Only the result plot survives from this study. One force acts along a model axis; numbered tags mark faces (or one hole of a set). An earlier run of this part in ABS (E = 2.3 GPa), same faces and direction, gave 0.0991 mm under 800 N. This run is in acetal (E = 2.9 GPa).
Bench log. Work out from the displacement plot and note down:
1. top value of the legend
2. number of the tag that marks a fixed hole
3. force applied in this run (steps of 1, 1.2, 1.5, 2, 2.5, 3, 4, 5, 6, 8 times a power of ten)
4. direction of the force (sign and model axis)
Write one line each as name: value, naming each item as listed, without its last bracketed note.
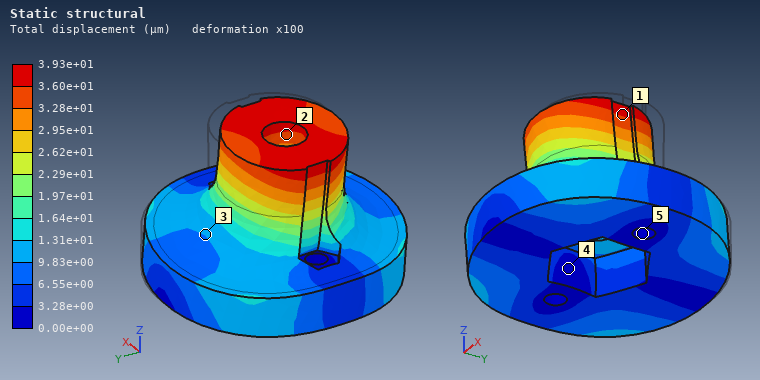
top value of the legend: 3.93e+01 µm
number of the tag that marks a fixed hole: 5
force applied in this run: 400 N
direction of the force: -X
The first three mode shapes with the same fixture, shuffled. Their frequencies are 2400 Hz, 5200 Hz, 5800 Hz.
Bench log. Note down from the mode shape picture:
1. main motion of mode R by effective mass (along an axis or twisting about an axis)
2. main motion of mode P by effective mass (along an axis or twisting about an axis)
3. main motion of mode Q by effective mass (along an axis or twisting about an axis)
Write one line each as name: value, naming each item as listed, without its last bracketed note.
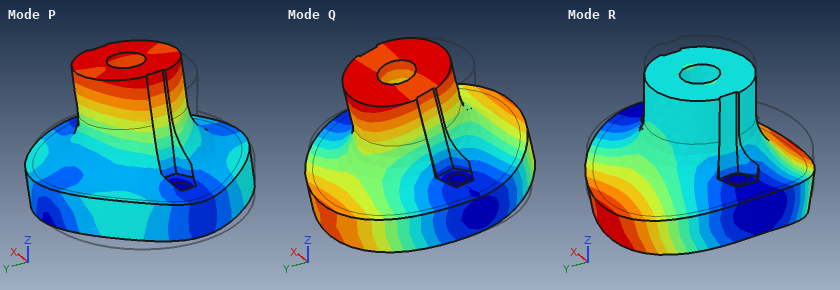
main motion of mode R by effective mass: along Z
main motion of mode P by effective mass: along X
main motion of mode Q by effective mass: along Y
